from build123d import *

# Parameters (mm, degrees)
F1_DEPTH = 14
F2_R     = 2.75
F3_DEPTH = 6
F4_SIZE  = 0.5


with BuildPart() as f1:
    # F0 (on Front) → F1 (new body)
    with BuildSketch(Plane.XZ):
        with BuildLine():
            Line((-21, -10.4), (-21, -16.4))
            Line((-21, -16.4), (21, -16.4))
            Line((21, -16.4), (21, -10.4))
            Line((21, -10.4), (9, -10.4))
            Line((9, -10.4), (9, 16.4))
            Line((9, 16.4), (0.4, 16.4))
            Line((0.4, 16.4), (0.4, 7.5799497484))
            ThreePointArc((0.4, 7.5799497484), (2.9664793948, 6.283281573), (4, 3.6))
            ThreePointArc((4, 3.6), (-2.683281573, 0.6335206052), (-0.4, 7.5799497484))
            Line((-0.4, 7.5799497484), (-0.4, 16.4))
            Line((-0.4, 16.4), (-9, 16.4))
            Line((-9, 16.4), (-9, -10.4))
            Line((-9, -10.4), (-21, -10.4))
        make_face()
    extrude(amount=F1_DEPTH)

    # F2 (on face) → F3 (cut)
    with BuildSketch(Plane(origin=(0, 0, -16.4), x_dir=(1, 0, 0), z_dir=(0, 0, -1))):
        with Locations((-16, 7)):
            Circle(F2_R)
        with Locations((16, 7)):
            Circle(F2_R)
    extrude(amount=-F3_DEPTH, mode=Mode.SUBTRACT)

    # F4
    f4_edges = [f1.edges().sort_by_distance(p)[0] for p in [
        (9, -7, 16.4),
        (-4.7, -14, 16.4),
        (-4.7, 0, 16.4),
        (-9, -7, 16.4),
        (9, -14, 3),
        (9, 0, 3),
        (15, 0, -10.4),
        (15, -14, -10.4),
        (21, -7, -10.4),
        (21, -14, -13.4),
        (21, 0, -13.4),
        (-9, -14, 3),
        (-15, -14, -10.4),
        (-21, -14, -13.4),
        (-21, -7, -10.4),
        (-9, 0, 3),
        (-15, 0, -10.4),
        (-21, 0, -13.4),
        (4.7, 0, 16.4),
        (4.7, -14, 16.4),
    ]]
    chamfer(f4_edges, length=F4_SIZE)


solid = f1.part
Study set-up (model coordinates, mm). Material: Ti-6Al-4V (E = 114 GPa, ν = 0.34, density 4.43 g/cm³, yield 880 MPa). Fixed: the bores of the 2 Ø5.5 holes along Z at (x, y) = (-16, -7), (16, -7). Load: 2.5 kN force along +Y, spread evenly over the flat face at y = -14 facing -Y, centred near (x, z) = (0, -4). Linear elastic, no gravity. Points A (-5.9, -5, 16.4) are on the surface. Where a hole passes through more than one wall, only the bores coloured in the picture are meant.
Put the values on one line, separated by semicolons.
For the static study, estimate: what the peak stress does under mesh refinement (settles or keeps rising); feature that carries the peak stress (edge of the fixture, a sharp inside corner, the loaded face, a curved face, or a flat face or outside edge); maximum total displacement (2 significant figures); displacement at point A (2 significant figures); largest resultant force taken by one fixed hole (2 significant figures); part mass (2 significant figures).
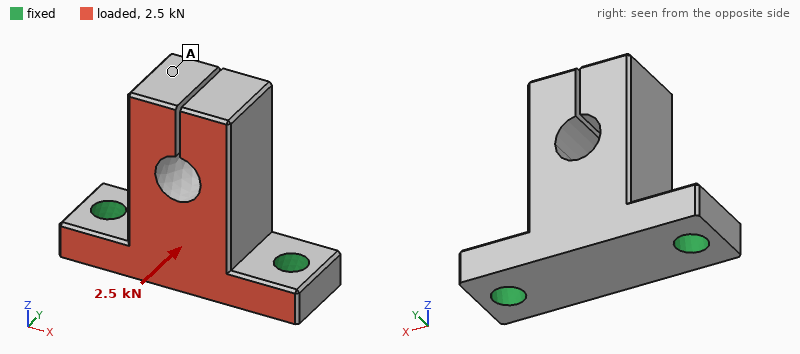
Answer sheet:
keeps rising; edge of the fixture; 90 µm; 87 µm; 1.3 kN; 41 g
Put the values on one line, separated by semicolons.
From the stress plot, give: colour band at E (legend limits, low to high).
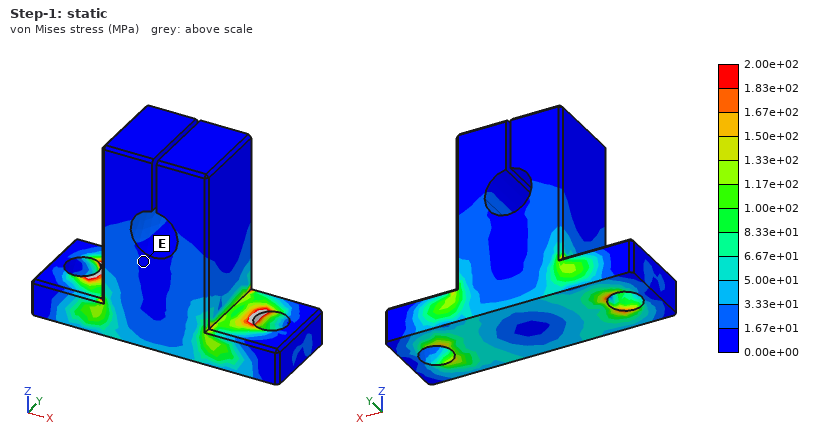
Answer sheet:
0.00e+00 to 1.67e+01 MPa
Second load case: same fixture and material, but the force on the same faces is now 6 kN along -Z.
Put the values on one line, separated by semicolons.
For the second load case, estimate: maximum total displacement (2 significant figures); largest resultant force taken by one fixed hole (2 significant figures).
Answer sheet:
0.13 mm; 3.1 kN
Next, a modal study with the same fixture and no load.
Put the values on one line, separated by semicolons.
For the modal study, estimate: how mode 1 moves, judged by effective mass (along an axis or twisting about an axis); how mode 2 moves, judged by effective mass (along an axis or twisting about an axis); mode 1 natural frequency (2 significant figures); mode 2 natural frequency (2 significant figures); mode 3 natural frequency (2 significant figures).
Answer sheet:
along Y; along X; 4900 Hz; 7800 Hz; 9500 Hz
